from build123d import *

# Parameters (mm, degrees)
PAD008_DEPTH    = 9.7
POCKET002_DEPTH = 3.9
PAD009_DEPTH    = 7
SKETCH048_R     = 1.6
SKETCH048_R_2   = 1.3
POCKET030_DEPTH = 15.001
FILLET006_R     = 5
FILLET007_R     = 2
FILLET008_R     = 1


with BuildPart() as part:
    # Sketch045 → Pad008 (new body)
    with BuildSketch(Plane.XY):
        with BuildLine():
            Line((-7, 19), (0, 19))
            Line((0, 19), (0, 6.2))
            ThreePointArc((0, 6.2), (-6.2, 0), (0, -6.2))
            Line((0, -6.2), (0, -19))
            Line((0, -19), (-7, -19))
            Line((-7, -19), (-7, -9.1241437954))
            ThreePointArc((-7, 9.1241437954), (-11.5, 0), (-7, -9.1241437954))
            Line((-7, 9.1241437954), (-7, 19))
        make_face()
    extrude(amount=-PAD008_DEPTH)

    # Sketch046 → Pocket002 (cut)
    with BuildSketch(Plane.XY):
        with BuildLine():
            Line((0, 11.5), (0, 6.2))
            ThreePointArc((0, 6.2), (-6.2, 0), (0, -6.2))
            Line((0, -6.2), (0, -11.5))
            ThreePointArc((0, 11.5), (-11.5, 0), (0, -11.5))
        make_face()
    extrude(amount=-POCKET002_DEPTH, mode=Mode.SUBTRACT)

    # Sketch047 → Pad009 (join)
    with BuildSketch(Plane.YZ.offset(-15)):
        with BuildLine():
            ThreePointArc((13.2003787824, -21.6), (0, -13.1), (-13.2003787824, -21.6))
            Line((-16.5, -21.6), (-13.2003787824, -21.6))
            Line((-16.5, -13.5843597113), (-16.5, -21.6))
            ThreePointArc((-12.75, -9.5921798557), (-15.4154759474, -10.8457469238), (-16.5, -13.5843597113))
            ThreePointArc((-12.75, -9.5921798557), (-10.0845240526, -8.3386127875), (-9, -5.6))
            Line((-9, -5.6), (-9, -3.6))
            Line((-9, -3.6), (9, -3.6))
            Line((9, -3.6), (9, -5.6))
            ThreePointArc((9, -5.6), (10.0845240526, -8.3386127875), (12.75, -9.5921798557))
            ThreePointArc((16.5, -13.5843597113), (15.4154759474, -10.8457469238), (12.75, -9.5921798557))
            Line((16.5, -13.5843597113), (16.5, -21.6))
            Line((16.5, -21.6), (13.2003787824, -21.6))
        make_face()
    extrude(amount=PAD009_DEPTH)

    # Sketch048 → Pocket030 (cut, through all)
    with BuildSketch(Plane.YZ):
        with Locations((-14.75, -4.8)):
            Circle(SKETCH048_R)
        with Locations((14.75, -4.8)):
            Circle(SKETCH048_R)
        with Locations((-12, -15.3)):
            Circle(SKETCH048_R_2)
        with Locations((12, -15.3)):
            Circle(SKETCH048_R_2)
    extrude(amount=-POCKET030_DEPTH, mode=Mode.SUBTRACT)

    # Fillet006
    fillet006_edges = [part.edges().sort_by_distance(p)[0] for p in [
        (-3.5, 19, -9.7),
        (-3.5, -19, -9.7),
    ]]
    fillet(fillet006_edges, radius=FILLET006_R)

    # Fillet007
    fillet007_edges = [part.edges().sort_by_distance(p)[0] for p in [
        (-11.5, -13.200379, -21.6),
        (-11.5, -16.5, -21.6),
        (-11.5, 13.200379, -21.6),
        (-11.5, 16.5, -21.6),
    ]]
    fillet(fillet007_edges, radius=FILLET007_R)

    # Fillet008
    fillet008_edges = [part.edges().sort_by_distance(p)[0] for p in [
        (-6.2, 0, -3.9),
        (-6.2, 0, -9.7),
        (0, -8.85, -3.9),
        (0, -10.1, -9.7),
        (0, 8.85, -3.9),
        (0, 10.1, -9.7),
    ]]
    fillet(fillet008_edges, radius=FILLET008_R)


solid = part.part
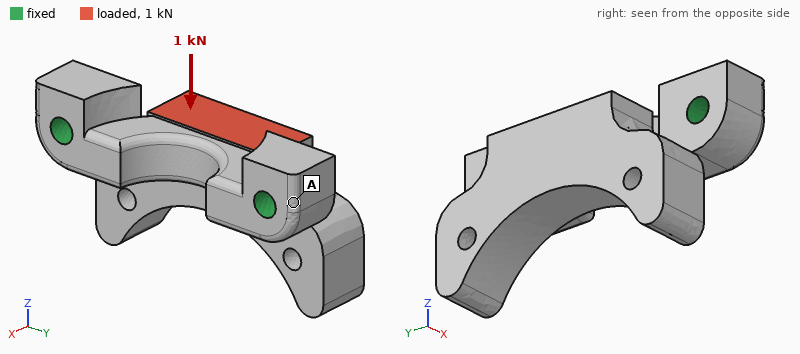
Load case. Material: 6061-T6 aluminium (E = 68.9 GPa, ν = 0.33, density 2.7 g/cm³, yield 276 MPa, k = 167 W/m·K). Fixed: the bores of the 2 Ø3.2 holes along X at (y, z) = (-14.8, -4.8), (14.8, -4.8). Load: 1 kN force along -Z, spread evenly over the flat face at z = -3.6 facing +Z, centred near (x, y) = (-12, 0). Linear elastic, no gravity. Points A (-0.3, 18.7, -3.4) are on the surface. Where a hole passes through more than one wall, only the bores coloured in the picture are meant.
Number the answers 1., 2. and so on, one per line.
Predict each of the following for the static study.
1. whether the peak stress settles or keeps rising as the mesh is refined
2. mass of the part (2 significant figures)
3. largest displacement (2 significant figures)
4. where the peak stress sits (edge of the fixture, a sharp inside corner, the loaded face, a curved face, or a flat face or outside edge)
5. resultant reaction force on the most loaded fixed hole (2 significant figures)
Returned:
1. keeps rising
2. 10 g
3. 0.10 mm
4. a sharp inside corner
5. 530 N
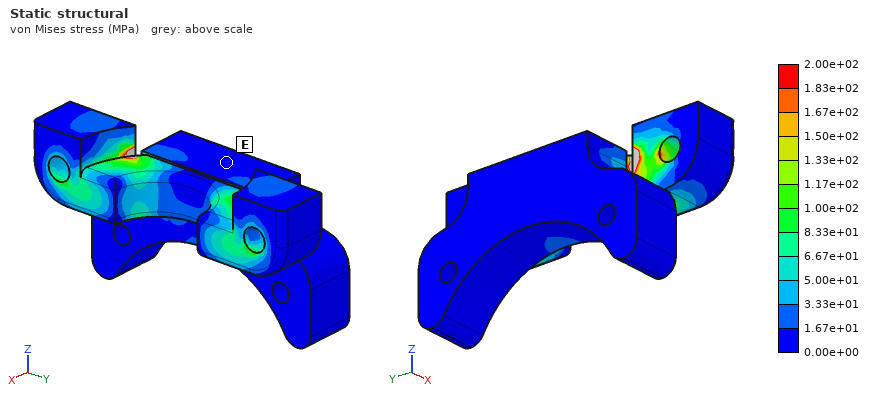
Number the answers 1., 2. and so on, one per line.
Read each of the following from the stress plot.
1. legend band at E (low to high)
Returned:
1. 0.00e+00 to 1.67e+01 MPa
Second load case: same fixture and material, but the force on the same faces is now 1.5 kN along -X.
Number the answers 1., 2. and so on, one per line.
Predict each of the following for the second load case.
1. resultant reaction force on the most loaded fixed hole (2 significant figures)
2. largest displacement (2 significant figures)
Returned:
1. 910 N
2. 60 µm
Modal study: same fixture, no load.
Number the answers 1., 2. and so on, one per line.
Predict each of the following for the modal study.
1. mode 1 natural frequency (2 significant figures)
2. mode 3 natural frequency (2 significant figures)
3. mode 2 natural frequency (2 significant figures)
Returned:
1. 6800 Hz
2. 14 kHz
3. 11 kHz
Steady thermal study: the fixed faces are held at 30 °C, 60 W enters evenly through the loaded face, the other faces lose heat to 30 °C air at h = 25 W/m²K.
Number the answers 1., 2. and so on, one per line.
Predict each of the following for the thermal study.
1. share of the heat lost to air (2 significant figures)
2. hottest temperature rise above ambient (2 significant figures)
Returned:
1. 3.1 %
2. 63 K
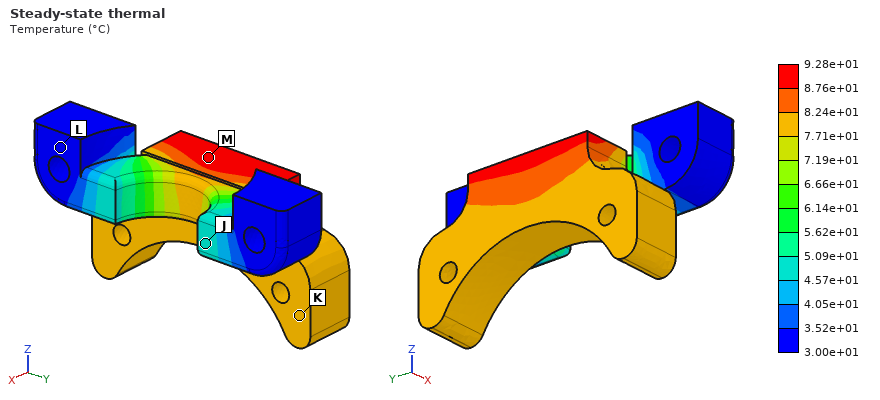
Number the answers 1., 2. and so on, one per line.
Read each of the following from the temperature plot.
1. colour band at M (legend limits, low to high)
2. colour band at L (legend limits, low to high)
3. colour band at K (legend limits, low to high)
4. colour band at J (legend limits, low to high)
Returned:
1. 8.76e+01 to 9.28e+01 °C
2. 3.00e+01 to 3.52e+01 °C
3. 7.71e+01 to 8.24e+01 °C
4. 4.57e+01 to 5.09e+01 °C
